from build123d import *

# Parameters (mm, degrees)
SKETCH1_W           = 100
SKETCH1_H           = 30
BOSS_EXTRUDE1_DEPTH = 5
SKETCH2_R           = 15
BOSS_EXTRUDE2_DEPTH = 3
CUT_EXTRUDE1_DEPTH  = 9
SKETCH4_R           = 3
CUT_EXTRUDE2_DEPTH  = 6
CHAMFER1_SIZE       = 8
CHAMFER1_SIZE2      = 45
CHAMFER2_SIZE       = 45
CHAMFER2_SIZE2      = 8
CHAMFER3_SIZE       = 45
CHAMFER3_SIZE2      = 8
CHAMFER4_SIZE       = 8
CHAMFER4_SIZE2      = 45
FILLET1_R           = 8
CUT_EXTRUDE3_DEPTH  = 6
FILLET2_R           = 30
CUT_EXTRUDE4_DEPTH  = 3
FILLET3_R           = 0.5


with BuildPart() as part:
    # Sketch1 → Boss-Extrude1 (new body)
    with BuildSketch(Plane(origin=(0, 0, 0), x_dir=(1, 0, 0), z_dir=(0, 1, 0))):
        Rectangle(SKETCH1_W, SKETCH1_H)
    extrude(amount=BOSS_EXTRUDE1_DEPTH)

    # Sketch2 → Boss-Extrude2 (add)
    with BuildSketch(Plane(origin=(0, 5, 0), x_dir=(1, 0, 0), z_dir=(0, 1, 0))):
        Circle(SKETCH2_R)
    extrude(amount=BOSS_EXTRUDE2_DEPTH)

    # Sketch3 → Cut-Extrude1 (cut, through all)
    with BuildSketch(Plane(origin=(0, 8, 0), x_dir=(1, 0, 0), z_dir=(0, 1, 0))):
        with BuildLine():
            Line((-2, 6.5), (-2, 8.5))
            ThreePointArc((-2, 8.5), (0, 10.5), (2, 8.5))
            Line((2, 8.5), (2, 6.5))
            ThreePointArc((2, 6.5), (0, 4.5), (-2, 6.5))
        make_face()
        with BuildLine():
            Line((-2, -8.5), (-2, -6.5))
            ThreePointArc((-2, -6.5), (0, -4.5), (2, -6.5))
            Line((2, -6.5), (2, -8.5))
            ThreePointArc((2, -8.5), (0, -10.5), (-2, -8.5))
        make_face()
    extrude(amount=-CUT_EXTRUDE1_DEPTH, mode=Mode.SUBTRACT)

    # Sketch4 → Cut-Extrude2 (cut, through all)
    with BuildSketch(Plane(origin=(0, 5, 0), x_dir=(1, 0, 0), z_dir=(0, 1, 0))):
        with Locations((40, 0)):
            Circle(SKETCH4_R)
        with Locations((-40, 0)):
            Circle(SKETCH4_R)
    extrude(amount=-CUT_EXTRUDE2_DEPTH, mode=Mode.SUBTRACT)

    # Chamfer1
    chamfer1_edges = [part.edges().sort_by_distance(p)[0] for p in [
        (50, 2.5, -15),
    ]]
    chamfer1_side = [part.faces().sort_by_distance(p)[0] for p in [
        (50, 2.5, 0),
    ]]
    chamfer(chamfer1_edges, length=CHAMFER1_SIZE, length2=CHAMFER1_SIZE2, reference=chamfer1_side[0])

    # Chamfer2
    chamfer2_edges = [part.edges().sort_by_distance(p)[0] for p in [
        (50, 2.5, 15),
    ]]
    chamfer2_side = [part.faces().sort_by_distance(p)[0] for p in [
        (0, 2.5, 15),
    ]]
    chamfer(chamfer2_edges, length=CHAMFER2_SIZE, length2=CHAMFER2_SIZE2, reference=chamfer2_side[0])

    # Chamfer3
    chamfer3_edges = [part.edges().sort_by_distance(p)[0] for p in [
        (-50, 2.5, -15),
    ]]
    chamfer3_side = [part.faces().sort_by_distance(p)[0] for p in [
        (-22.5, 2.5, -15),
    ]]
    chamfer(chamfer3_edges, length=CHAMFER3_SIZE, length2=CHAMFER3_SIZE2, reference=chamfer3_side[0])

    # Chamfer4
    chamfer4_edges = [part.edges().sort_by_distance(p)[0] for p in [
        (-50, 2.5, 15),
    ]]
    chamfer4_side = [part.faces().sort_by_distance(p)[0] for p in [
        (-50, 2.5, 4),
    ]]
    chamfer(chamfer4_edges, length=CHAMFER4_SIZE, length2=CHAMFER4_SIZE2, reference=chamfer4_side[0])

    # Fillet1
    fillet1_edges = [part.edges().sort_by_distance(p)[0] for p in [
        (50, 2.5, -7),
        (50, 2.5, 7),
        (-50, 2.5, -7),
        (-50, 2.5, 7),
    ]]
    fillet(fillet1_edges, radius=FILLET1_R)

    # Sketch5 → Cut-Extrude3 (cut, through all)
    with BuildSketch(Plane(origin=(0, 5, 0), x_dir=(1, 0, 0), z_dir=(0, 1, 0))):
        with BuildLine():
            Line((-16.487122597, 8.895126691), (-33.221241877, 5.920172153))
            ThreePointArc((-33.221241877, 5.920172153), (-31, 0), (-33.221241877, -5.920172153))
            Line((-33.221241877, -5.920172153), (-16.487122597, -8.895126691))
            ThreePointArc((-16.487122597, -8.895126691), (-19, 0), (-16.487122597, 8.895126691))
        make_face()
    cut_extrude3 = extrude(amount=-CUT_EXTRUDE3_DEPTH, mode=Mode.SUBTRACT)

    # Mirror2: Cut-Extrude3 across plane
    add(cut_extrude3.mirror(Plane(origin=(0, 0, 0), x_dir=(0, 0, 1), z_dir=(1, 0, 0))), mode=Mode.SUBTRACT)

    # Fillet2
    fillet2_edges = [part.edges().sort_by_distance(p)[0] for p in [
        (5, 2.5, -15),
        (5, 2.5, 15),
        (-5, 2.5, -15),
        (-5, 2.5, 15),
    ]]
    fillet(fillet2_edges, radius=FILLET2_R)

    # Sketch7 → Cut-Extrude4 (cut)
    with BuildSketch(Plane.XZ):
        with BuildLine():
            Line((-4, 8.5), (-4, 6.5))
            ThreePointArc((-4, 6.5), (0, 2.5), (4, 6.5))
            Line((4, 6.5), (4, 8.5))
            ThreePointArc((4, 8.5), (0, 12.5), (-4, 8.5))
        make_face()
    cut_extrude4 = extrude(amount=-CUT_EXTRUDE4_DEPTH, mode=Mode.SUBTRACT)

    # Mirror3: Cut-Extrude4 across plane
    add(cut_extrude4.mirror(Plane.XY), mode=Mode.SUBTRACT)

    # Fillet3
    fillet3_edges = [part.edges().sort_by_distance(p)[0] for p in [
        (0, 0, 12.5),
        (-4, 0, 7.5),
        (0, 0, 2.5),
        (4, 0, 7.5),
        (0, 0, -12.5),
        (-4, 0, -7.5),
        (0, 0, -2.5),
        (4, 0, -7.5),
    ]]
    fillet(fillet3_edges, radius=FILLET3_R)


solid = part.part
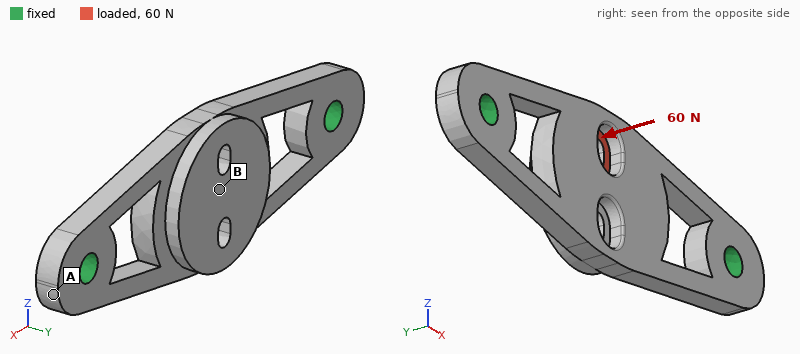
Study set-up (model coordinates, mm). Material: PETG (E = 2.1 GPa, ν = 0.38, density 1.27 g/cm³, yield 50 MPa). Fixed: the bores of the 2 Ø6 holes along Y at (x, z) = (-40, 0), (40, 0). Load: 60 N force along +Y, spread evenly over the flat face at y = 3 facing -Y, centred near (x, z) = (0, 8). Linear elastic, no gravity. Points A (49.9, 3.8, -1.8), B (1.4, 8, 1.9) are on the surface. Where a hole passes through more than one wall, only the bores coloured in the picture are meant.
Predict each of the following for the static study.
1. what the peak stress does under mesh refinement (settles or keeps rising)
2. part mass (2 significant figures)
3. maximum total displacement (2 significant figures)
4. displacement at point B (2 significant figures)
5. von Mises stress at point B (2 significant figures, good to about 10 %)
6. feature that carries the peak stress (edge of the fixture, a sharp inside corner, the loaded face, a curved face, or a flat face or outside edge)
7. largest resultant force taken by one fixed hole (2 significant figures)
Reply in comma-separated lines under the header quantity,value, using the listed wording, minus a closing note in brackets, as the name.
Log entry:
quantity,value
what the peak stress does under mesh refinement,keeps rising
part mass,13 g
maximum total displacement,0.64 mm
displacement at point B,0.39 mm
von Mises stress at point B,3.9 MPa
feature that carries the peak stress,a sharp inside corner
largest resultant force taken by one fixed hole,34 N
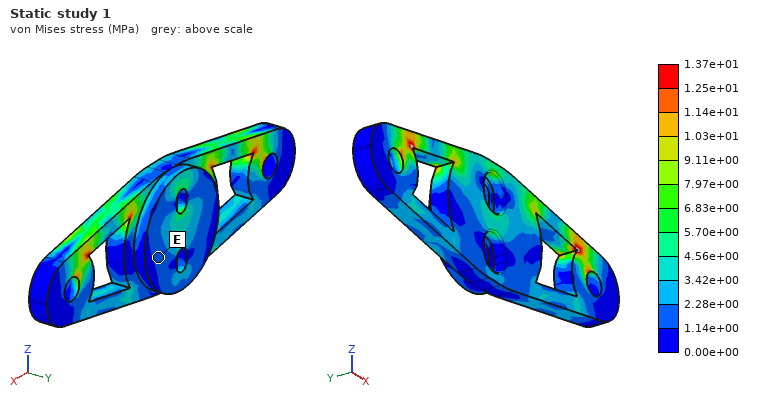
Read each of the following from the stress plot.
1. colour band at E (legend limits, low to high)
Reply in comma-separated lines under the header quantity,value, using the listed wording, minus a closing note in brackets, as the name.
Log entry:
quantity,value
colour band at E,1.14e+00 to 2.28e+00 MPa
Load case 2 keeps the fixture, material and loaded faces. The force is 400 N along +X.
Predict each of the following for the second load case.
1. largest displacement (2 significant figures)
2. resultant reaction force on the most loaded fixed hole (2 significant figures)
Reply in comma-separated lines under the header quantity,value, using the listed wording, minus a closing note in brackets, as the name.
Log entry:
quantity,value
largest displacement,0.13 mm
resultant reaction force on the most loaded fixed hole,200 N
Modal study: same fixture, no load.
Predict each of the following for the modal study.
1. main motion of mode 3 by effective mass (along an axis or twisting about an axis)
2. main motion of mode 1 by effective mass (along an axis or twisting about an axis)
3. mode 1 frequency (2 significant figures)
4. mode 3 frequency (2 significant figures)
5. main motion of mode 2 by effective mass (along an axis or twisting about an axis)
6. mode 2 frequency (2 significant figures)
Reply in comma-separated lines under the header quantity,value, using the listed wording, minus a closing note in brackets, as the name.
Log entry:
quantity,value
main motion of mode 3 by effective mass,along Z
main motion of mode 1 by effective mass,along Y
mode 1 frequency,750 Hz
mode 3 frequency,1100 Hz
main motion of mode 2 by effective mass,along Z
mode 2 frequency,940 Hz
